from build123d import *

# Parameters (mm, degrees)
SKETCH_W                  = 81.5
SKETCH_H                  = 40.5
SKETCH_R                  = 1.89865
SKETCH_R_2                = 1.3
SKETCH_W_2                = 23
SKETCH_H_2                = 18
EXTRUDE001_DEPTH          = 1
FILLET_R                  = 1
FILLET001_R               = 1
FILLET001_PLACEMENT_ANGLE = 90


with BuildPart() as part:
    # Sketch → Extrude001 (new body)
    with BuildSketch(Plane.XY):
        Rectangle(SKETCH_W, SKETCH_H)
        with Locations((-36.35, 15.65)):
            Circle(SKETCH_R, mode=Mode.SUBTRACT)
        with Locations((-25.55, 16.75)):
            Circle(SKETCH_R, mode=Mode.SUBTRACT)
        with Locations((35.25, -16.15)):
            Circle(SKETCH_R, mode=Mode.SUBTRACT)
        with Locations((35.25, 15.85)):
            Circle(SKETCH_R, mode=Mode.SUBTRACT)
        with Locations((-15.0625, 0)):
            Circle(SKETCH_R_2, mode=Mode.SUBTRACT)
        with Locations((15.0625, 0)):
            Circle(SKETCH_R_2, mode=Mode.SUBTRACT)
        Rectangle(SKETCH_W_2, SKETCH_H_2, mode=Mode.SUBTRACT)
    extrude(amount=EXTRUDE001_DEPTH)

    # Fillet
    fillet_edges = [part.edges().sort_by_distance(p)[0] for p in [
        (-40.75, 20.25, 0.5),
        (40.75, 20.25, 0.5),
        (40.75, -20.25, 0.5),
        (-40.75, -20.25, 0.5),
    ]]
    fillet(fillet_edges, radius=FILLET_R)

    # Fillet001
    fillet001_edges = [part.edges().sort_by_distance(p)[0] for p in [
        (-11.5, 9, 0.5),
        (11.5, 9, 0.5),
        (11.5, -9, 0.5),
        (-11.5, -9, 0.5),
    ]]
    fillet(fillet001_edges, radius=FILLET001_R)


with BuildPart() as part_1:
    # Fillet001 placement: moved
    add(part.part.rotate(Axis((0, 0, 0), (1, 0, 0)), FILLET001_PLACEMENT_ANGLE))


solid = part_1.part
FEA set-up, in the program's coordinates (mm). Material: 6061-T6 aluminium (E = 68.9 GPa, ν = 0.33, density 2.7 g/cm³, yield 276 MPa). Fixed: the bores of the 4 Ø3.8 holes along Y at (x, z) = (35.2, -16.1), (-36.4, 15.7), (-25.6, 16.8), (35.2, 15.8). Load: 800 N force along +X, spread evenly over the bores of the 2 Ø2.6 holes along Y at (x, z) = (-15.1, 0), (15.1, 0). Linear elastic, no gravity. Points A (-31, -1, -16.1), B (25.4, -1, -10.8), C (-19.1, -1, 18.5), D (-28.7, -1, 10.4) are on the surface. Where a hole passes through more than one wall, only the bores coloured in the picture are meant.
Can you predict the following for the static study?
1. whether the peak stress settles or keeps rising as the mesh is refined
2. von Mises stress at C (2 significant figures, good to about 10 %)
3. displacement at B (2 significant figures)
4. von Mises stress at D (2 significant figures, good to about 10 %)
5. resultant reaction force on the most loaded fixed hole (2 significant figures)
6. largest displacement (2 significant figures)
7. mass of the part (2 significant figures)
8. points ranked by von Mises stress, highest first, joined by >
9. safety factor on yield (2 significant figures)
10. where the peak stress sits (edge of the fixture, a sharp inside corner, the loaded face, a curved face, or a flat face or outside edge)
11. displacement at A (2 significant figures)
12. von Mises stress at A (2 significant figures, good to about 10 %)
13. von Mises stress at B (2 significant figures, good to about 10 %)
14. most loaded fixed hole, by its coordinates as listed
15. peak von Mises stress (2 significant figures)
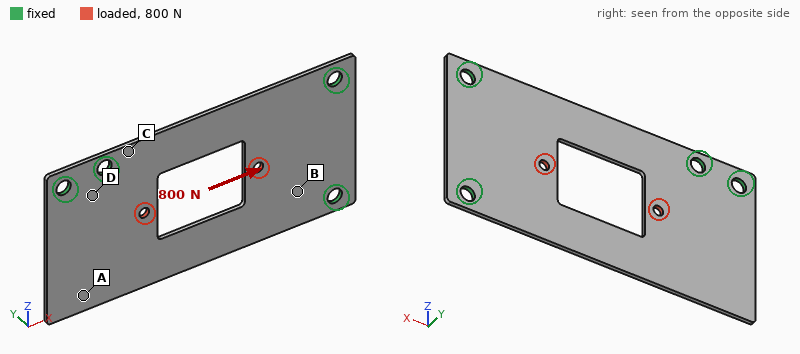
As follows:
settles
13 MPa
4.2 µm
26 MPa
280 N
16 µm
7.6 g
D > B > C > A
2.5
the loaded face
11 µm
5.4 MPa
19 MPa
(35.2, -16.1)
110 MPa
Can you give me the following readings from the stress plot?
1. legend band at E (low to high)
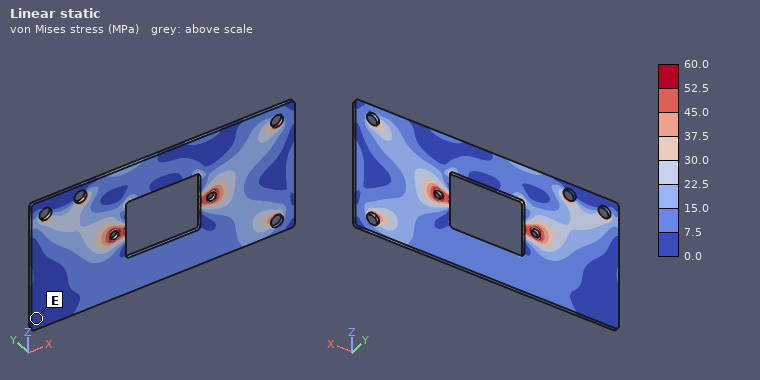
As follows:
0.0 to 7.5 MPa
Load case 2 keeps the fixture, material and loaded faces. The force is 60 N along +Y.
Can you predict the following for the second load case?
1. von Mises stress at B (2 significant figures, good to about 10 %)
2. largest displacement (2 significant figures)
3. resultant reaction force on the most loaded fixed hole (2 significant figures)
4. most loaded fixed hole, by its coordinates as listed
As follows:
28 MPa
0.57 mm
38 N
(-25.6, 16.8)
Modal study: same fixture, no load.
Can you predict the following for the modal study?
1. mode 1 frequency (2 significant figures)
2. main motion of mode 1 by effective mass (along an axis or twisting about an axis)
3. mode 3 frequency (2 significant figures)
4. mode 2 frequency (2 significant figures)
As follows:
700 Hz
along Y
1900 Hz
1300 Hz
